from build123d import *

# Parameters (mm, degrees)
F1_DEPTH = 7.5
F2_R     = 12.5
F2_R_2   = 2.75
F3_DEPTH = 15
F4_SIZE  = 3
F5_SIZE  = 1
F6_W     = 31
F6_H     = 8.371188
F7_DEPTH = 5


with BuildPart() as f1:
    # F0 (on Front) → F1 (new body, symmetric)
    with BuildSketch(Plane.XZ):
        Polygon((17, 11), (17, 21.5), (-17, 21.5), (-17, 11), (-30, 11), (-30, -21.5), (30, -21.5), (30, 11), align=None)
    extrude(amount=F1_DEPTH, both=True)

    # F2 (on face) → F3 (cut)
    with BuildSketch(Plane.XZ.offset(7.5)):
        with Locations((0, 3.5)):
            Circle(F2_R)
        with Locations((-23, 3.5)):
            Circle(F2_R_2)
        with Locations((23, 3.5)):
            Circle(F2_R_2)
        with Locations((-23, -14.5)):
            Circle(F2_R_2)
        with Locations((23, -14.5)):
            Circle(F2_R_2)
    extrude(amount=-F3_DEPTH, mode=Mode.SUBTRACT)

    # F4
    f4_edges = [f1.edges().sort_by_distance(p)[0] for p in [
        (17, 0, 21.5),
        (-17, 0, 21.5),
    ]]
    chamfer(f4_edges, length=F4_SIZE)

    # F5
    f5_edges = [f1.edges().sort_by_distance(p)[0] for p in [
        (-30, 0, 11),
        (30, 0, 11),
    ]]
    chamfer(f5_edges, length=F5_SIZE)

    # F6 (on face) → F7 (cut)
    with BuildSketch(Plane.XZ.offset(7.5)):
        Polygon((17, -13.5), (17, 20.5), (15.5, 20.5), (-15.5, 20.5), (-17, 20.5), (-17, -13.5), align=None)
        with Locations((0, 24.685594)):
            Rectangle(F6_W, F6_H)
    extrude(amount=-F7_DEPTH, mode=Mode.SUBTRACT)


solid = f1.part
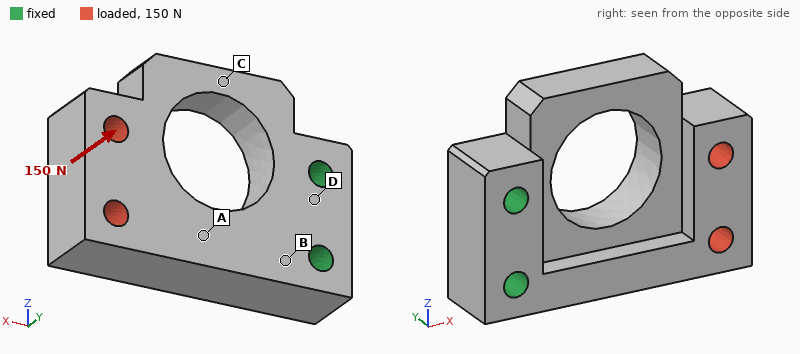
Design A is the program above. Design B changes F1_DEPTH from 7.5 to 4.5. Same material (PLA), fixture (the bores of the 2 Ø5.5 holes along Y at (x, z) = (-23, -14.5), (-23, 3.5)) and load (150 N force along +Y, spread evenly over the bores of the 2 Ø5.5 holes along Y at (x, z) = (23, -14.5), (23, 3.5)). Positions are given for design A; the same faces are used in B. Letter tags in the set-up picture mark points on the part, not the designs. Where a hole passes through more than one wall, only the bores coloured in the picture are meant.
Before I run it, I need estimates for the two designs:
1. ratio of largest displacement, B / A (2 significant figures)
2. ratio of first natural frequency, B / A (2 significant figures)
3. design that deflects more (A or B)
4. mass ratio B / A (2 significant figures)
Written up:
3.4
0.69
B
0.63
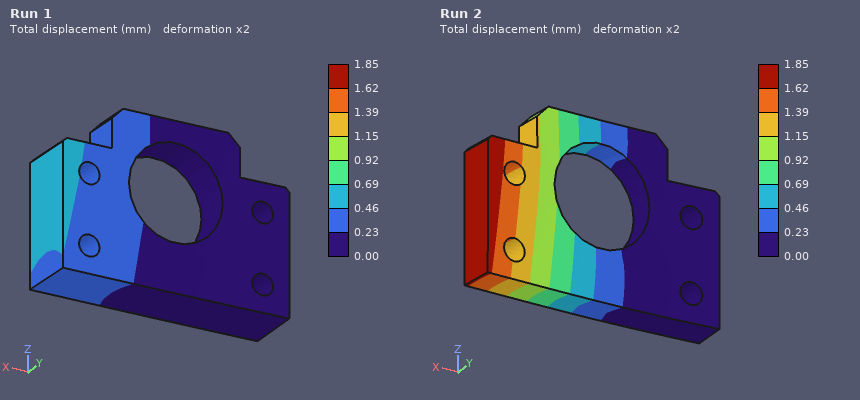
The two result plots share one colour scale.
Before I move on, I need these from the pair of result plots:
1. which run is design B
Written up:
Run 2
